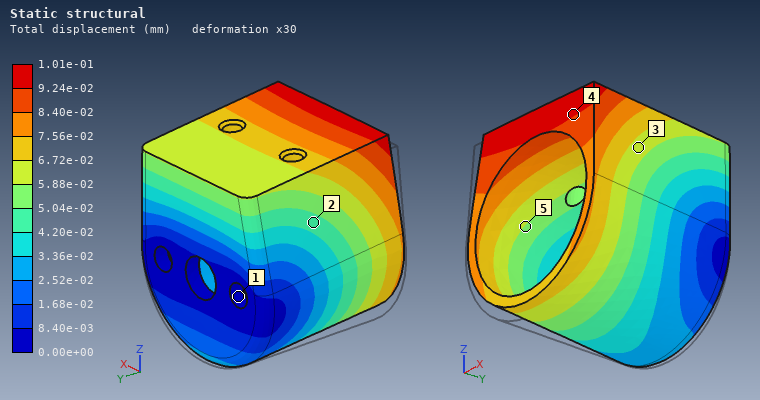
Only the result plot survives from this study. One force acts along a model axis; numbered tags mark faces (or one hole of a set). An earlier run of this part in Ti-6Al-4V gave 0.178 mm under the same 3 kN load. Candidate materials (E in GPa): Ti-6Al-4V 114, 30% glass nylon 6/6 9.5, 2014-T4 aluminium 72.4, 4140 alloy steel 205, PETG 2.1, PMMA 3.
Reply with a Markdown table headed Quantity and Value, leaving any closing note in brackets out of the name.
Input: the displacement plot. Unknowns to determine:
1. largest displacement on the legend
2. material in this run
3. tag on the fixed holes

| Quantity | Value |
|---|---|
| largest displacement on the legend | 1.01e-01 mm |
| material in this run | 4140 alloy steel |
| tag on the fixed holes | 1 |
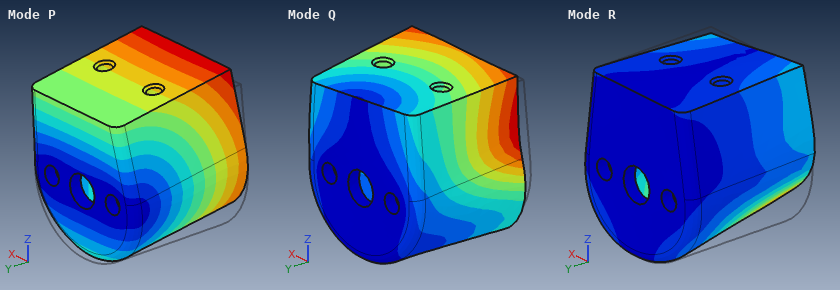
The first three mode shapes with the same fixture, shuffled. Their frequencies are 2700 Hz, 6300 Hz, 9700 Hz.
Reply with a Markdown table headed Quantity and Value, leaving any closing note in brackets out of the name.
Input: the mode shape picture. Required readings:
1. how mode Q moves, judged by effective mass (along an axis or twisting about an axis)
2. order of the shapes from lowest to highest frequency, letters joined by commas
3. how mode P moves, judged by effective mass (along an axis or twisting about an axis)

| Quantity | Value |
|---|---|
| how mode Q moves, judged by effective mass | along X |
| order of the shapes from lowest to highest frequency, letters joined by commas | P, Q, R |
| how mode P moves, judged by effective mass | along Z |
